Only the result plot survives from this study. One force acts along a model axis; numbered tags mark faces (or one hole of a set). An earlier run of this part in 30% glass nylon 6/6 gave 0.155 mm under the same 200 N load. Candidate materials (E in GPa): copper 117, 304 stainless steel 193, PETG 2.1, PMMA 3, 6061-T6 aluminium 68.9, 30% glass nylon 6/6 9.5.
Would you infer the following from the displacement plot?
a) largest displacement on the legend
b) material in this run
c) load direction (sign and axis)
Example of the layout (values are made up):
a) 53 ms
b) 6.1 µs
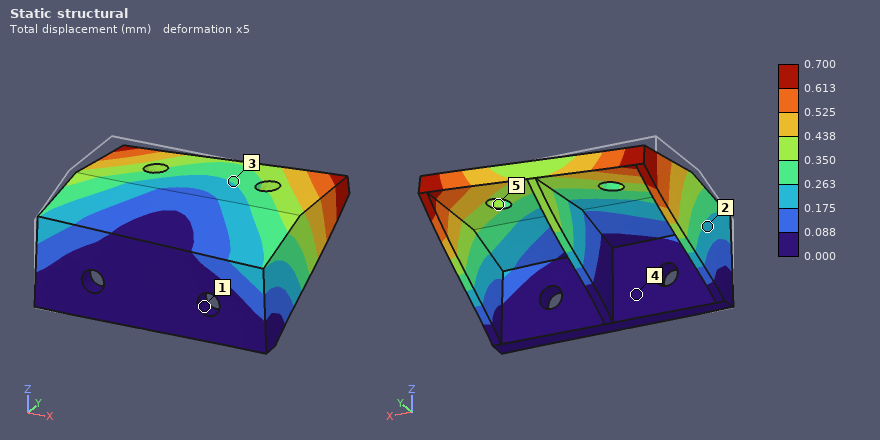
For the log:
a) 0.700 mm
b) PETG
c) +X
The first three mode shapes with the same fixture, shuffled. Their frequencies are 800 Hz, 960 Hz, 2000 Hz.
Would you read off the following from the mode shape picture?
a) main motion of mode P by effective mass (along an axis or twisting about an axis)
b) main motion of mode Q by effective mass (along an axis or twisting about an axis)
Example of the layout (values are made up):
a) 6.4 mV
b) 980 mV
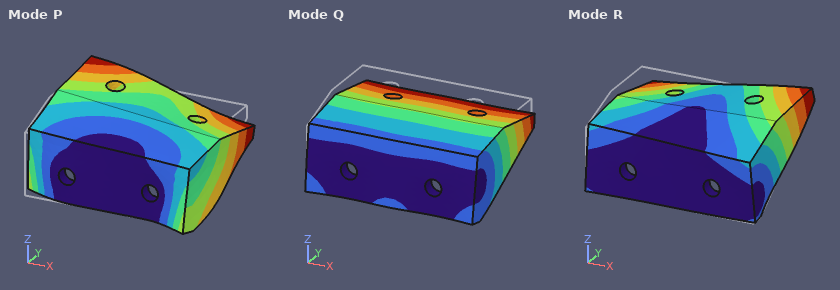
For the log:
a) along X
b) along Z
